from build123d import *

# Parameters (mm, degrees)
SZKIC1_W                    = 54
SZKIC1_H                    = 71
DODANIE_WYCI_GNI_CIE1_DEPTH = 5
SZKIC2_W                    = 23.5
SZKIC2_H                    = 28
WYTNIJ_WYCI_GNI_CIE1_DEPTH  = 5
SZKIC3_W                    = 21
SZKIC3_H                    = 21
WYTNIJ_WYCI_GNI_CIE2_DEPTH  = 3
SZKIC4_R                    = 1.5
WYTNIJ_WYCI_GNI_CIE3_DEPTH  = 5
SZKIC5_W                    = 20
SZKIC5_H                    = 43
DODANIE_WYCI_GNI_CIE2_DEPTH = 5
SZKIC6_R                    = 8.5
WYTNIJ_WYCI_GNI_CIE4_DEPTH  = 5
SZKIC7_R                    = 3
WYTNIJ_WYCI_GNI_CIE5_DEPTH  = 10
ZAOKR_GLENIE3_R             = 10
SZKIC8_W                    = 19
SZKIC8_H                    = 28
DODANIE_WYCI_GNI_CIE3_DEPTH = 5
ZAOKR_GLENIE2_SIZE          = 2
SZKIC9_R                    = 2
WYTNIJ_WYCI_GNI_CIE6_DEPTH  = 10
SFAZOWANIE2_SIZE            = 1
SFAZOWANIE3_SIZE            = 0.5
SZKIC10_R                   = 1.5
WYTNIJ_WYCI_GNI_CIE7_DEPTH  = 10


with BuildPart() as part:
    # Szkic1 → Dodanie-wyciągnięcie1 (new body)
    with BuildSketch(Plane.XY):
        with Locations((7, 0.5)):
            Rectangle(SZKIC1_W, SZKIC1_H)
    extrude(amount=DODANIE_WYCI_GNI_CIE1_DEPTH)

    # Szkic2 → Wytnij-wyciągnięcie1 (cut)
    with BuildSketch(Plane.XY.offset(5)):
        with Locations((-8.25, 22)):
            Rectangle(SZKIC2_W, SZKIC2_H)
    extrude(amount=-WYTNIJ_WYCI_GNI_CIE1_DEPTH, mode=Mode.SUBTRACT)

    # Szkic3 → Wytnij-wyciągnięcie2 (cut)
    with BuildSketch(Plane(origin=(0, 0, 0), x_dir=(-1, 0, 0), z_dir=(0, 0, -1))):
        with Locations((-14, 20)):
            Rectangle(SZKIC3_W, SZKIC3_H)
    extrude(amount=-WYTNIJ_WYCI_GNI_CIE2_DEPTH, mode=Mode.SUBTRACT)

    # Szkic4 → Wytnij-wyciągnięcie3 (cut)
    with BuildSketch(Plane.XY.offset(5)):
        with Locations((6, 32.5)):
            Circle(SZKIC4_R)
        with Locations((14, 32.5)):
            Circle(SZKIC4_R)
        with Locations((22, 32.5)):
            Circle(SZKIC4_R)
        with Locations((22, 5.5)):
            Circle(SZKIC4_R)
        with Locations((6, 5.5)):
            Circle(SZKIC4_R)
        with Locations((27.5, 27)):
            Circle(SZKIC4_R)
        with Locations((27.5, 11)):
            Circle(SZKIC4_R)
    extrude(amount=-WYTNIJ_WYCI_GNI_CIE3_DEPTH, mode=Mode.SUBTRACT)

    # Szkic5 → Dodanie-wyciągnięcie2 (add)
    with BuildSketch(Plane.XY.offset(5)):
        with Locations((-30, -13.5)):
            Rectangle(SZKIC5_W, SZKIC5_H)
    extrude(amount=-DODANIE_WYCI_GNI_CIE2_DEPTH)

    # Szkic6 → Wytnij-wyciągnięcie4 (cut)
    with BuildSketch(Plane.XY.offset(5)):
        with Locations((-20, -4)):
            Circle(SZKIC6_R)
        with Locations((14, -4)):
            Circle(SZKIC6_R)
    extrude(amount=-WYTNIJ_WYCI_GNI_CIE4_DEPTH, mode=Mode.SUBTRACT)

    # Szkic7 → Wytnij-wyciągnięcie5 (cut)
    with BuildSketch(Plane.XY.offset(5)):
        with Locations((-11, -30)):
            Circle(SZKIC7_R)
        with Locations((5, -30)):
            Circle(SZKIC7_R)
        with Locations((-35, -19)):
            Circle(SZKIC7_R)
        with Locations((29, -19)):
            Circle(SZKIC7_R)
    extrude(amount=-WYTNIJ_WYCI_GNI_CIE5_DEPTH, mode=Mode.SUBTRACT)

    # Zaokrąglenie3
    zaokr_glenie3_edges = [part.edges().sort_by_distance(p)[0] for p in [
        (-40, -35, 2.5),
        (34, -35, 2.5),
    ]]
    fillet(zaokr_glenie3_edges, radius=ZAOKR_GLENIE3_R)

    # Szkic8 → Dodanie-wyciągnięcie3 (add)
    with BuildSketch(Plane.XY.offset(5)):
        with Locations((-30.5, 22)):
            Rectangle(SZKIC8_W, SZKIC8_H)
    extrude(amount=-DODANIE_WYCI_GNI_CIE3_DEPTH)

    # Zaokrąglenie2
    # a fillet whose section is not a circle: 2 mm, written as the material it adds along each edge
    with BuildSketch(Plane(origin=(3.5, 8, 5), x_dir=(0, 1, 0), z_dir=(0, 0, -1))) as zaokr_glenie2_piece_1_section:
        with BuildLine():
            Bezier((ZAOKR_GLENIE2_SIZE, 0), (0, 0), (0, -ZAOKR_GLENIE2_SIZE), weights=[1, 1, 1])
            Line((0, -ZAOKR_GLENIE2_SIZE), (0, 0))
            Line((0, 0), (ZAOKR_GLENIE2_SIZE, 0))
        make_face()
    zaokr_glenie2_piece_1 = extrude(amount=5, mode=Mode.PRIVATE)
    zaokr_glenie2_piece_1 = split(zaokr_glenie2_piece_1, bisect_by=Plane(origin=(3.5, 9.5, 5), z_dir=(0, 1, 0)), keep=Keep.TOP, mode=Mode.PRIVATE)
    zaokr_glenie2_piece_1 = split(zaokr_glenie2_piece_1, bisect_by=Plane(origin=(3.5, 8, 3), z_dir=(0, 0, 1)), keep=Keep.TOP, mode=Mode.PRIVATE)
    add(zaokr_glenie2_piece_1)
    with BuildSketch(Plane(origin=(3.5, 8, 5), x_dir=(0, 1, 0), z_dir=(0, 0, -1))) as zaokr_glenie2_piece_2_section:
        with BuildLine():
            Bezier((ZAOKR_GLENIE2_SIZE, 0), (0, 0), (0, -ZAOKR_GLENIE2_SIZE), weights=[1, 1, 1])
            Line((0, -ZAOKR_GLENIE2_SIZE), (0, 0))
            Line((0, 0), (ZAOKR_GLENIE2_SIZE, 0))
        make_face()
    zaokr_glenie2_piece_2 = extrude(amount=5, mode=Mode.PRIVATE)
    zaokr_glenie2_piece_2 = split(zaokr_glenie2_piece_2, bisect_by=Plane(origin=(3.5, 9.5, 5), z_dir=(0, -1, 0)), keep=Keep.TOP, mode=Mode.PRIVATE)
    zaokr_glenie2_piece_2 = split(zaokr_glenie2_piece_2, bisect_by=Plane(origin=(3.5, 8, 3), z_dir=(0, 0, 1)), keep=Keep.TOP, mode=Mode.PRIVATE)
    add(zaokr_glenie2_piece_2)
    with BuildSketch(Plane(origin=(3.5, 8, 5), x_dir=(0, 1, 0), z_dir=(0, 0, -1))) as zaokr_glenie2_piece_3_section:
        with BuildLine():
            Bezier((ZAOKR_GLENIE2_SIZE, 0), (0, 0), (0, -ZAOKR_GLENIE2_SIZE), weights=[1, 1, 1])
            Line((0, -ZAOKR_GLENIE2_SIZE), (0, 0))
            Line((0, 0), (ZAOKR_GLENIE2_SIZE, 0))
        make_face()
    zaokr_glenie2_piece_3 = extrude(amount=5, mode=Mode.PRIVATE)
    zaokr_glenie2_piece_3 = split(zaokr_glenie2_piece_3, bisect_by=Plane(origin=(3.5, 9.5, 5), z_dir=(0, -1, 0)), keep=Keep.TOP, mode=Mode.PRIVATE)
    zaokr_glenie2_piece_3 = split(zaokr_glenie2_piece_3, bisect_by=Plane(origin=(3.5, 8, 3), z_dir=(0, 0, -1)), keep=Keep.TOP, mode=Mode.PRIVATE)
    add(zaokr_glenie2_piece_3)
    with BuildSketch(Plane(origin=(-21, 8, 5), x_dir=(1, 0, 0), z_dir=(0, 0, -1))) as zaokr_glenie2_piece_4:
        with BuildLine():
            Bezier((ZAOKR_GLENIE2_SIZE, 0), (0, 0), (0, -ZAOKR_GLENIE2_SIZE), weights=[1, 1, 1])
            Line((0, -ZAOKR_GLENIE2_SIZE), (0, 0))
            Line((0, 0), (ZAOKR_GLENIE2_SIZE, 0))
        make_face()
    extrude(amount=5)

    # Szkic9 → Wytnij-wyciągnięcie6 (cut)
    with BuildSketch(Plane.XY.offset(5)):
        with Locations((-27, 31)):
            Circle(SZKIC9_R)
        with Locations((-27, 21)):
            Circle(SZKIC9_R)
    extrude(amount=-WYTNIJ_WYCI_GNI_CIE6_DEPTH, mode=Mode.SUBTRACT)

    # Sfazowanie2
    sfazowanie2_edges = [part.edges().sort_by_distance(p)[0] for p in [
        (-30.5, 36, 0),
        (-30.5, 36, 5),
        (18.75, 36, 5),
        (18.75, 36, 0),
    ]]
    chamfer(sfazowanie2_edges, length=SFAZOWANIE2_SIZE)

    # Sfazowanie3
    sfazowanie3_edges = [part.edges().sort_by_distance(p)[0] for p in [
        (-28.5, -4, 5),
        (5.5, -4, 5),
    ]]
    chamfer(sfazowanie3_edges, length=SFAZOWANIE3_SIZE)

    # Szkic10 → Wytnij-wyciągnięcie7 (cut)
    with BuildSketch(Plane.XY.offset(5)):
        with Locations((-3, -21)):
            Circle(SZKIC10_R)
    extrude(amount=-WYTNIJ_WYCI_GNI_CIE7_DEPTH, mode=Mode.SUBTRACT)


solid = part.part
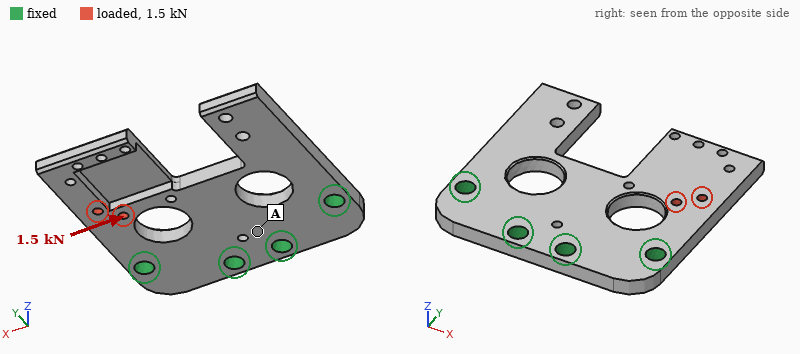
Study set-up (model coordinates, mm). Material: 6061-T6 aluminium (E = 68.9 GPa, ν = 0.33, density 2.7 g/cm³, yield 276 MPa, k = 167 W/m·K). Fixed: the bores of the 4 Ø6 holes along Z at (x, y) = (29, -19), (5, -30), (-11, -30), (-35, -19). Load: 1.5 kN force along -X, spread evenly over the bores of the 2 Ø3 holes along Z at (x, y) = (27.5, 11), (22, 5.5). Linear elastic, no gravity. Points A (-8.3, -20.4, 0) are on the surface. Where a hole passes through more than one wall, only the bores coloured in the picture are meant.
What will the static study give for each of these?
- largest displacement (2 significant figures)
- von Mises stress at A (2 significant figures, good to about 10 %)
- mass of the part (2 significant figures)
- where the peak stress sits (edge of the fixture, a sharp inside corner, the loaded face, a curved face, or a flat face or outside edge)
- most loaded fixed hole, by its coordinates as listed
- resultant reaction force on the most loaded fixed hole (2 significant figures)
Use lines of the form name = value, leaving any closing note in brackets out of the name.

largest displacement = 33 µm
von Mises stress at A = 7.9 MPa
mass of the part = 49 g
where the peak stress sits = a curved face
most loaded fixed hole, by its coordinates as listed = (29, -19)
resultant reaction force on the most loaded fixed hole = 1.0 kN
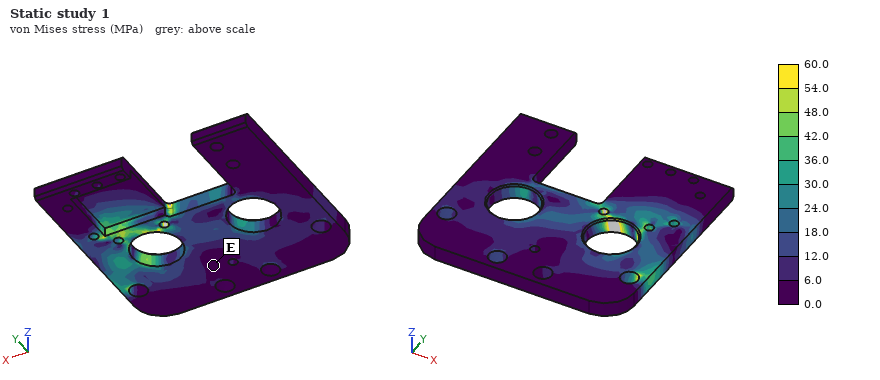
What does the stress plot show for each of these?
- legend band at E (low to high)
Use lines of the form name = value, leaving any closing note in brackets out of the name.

legend band at E = 0.0 to 6.0 MPa
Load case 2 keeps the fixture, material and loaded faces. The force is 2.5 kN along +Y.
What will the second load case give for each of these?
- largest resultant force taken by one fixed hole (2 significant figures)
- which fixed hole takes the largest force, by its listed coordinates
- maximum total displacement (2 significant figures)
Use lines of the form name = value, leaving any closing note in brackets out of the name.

largest resultant force taken by one fixed hole = 2.1 kN
which fixed hole takes the largest force, by its listed coordinates = (29, -19)
maximum total displacement = 21 µm
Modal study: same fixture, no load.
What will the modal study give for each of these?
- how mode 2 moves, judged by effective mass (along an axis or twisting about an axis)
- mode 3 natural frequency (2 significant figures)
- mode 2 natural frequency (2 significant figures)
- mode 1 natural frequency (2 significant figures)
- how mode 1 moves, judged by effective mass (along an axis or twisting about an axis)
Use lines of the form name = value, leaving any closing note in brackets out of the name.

how mode 2 moves, judged by effective mass = twisting about Y
mode 3 natural frequency = 4200 Hz
mode 2 natural frequency = 1600 Hz
mode 1 natural frequency = 1400 Hz
how mode 1 moves, judged by effective mass = along Z
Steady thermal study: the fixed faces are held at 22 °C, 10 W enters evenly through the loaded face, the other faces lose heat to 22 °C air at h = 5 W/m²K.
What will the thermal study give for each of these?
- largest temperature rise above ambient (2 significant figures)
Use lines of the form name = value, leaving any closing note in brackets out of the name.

largest temperature rise above ambient = 17 K
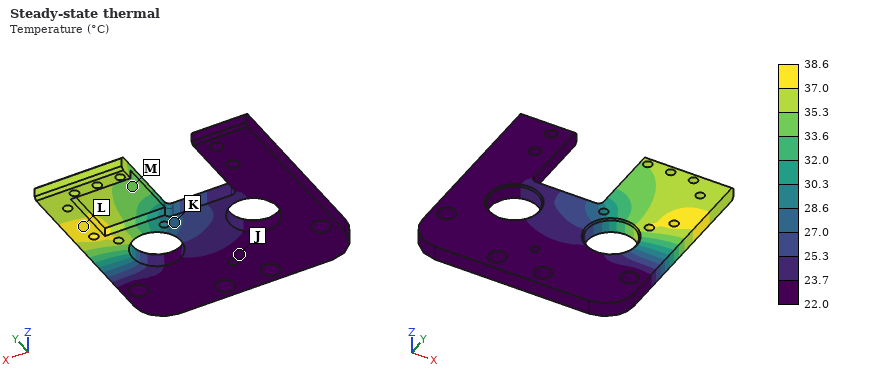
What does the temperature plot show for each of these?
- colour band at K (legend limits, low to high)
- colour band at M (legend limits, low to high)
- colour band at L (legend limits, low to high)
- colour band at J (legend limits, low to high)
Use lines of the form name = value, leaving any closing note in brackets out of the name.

colour band at K = 27.0 to 28.6 °C
colour band at M = 33.6 to 35.3 °C
colour band at L = 37.0 to 38.6 °C
colour band at J = 22.0 to 23.7 °C
